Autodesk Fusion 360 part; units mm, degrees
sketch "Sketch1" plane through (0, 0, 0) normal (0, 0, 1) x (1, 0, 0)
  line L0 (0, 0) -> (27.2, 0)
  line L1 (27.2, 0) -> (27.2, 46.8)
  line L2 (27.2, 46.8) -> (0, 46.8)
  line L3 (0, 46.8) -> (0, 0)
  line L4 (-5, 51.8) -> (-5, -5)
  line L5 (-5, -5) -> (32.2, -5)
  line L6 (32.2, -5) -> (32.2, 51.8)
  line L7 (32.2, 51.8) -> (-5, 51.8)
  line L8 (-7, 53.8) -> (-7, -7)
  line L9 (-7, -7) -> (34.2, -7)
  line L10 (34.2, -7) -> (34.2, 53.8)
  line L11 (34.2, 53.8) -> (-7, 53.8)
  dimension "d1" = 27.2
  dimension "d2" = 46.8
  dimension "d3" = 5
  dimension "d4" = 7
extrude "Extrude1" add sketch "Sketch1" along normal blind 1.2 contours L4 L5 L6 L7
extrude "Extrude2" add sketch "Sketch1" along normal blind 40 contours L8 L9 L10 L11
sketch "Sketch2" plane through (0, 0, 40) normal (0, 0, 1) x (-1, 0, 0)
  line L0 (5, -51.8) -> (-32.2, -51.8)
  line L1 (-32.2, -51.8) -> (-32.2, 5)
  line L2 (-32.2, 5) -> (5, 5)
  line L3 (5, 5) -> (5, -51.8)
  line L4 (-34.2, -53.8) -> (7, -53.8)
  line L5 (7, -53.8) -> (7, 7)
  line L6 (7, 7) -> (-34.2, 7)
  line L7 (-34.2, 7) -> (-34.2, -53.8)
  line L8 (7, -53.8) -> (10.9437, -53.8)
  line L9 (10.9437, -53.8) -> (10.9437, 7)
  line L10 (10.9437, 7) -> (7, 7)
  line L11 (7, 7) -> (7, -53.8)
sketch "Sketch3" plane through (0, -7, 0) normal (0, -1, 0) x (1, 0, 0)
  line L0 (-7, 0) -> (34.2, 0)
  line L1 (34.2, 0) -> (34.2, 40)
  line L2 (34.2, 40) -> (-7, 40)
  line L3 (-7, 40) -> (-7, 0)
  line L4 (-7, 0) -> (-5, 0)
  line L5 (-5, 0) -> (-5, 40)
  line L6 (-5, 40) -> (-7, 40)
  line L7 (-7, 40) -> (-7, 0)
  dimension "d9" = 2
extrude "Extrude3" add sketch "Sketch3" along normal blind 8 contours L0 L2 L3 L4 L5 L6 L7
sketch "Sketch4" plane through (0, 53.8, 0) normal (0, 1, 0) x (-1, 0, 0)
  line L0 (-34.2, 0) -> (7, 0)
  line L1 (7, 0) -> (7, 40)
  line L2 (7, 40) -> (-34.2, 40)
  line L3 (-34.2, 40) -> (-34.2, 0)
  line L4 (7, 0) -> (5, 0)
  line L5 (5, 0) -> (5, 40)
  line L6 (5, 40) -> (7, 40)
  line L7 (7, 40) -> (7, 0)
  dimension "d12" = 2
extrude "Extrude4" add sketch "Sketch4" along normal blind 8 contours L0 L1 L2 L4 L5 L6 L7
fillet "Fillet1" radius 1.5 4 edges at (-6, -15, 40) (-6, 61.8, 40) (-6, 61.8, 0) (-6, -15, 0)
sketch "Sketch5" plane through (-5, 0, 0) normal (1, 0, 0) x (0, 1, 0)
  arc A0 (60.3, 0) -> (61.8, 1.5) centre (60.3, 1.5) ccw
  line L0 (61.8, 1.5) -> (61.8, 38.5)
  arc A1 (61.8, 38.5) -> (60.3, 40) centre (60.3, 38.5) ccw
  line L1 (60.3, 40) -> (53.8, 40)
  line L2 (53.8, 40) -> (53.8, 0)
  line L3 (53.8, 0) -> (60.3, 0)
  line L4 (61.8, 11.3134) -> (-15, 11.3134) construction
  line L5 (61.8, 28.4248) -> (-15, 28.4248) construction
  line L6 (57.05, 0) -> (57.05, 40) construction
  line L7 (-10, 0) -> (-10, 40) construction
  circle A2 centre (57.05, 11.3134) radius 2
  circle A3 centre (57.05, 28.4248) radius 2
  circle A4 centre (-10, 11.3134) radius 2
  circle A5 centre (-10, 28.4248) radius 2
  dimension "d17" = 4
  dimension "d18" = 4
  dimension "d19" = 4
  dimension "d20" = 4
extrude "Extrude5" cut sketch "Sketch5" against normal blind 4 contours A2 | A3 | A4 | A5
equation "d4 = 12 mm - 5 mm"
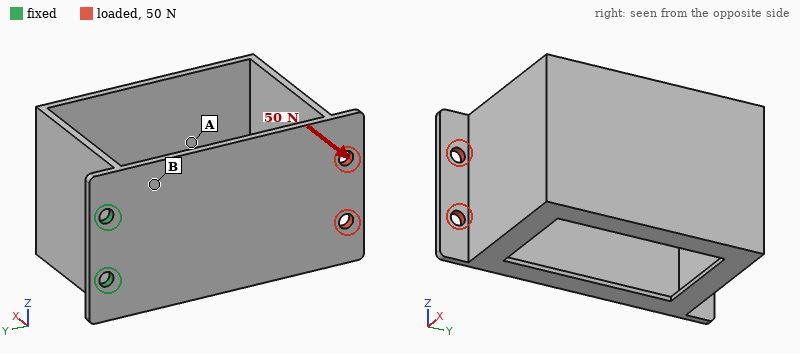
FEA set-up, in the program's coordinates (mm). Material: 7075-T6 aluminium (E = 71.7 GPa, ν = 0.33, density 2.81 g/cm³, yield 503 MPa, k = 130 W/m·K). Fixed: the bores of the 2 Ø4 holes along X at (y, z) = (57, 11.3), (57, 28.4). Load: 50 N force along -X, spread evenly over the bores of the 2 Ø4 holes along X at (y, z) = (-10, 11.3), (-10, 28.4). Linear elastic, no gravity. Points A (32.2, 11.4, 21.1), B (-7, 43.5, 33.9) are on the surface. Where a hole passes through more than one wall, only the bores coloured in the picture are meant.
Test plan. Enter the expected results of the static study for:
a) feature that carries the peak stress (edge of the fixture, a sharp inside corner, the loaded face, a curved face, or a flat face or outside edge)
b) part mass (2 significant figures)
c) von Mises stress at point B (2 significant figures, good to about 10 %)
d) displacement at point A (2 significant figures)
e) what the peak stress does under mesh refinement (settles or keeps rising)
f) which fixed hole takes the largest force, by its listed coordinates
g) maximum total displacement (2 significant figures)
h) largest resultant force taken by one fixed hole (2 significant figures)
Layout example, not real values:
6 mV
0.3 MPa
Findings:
edge of the fixture
50 g
34 MPa
0.74 mm
keeps rising
(57, 11.3)
0.96 mm
37 N
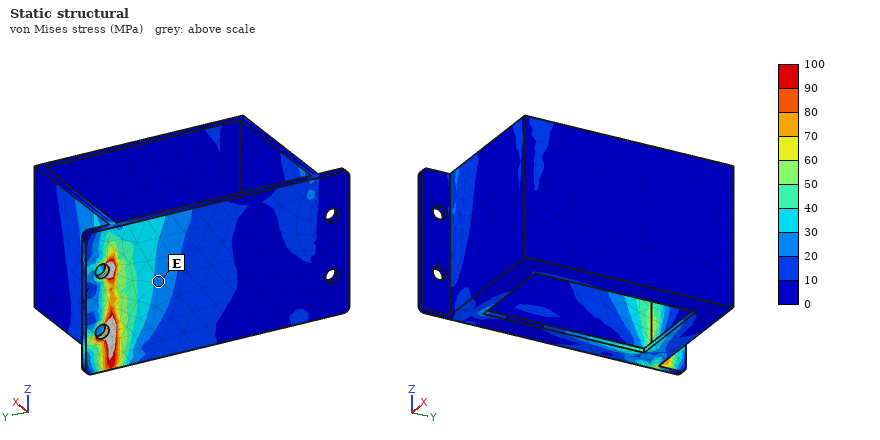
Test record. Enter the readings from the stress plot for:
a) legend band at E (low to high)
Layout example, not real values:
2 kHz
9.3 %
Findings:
20 to 30 MPa
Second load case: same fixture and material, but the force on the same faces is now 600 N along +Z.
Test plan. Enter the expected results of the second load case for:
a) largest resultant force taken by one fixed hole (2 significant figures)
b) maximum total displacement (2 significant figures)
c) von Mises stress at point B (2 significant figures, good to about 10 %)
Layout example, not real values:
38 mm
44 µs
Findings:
2.0 kN
0.18 mm
42 MPa
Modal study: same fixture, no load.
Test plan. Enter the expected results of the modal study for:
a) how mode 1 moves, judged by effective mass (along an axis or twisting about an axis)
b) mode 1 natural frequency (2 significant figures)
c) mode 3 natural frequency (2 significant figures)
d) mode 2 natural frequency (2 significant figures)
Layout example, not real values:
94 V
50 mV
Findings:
along X
250 Hz
1600 Hz
710 Hz
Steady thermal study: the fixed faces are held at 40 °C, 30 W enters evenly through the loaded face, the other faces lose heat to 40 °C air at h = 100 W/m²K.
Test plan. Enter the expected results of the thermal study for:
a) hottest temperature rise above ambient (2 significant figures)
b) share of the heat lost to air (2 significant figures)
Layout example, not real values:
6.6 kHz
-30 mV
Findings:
63 K
87 %
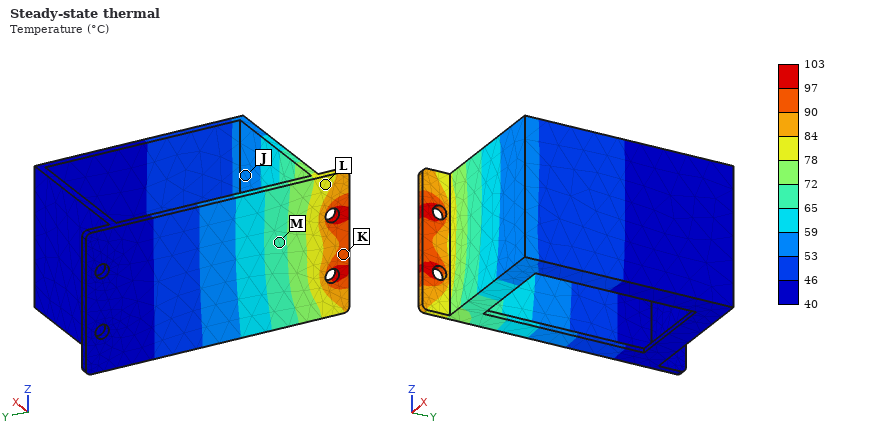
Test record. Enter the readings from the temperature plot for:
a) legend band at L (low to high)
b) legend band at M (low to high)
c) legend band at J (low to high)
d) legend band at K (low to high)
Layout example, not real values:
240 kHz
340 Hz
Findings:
78 to 84 °C
65 to 72 °C
53 to 59 °C
90 to 97 °C
